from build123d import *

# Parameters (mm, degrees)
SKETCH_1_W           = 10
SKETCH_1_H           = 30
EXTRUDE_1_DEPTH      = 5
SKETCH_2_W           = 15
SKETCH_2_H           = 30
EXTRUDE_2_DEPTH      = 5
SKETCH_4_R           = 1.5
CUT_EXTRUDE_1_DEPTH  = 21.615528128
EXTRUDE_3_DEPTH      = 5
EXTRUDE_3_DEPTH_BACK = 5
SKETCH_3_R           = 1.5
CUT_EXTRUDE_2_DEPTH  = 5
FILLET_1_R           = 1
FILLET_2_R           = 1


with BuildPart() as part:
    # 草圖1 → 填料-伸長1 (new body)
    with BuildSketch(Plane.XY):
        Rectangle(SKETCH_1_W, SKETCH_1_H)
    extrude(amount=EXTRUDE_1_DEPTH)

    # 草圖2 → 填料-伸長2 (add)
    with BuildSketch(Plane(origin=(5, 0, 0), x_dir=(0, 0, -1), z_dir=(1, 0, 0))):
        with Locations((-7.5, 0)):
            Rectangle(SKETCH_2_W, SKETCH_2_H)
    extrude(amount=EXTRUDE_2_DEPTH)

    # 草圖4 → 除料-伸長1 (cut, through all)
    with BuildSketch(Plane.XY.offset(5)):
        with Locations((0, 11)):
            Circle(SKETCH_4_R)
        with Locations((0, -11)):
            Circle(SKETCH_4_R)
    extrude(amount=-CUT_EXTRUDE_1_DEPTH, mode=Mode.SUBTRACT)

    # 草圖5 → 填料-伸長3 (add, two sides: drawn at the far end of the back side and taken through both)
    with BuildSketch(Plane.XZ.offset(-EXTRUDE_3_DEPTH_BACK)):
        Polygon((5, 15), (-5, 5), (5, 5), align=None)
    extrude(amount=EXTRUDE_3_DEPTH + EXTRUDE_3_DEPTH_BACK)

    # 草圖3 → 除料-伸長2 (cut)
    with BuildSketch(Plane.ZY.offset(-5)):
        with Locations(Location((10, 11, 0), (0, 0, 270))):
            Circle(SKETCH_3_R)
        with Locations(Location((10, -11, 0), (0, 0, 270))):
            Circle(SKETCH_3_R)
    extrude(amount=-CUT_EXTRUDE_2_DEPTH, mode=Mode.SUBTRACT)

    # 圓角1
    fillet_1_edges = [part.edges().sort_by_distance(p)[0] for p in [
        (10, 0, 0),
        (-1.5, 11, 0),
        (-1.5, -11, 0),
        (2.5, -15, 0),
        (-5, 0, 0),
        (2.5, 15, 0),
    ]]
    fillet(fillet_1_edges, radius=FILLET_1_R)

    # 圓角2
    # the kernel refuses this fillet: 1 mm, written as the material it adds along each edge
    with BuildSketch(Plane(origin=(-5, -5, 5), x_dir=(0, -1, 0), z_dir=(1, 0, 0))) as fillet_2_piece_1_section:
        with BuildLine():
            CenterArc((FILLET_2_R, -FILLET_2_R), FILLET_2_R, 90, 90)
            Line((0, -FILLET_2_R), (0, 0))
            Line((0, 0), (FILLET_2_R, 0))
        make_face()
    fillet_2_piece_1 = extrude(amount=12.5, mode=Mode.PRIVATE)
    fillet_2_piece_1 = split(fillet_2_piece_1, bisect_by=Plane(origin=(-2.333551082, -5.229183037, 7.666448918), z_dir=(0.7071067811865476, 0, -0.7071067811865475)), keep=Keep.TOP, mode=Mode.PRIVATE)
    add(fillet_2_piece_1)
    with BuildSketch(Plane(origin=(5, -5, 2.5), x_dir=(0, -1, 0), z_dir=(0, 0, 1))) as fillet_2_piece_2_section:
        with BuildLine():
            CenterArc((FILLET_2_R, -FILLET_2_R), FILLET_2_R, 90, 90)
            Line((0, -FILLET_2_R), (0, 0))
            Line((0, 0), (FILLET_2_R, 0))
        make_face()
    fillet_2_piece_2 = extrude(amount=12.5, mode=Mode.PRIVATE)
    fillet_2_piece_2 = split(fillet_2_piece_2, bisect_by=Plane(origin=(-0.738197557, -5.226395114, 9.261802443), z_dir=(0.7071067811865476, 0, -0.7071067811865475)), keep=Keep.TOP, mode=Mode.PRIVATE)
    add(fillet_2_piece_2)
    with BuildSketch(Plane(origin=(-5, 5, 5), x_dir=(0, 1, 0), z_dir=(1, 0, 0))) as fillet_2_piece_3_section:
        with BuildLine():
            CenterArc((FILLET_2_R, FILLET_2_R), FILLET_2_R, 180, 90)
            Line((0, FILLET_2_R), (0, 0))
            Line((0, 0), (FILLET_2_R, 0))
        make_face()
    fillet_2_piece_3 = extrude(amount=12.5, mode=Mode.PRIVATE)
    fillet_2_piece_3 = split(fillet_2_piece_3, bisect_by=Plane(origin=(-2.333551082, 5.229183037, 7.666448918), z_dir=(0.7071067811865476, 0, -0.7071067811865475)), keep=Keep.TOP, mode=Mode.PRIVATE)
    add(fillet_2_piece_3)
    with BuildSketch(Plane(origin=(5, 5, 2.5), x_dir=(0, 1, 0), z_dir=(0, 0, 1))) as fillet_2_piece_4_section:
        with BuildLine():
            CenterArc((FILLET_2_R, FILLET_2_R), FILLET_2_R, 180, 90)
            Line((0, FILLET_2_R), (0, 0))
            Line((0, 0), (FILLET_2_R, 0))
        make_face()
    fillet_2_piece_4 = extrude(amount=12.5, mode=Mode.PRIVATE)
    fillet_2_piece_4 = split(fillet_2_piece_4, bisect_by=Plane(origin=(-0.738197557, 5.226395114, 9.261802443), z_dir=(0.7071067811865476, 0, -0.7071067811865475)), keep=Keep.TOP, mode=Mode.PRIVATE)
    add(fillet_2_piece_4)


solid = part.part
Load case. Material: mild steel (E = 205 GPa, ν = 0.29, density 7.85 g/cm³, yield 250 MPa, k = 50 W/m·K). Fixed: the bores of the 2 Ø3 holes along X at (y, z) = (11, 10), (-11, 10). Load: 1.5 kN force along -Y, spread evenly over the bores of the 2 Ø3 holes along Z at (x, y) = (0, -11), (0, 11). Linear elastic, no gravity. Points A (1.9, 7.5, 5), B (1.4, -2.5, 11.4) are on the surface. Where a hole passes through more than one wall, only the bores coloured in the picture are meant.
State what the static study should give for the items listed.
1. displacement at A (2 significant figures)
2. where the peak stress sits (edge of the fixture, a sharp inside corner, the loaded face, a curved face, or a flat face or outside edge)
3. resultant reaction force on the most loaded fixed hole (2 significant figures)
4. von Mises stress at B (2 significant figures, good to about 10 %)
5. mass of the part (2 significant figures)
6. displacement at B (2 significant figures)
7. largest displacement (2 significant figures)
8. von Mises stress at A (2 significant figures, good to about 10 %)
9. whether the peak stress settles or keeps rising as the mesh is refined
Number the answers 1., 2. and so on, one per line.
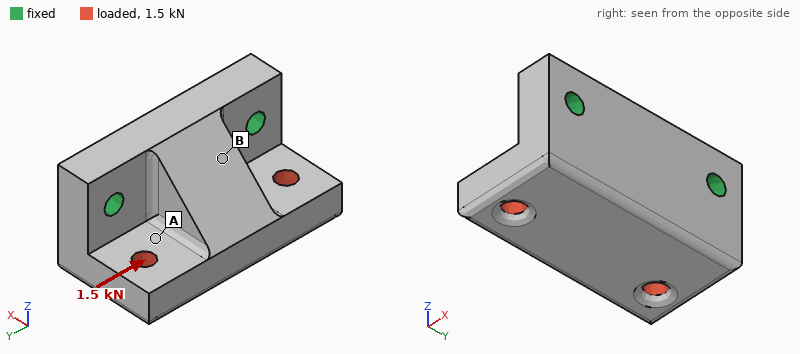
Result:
1. 2.2 µm
2. edge of the fixture
3. 1.0 kN
4. 13 MPa
5. 32 g
6. 1.1 µm
7. 4.0 µm
8. 26 MPa
9. keeps rising
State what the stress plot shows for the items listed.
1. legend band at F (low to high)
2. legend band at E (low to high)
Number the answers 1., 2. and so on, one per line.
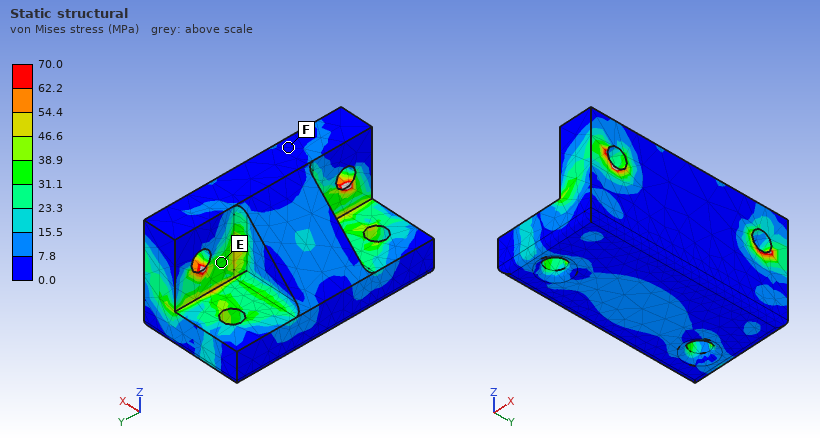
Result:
1. 0.0 to 7.8 MPa
2. 31.1 to 38.9 MPa
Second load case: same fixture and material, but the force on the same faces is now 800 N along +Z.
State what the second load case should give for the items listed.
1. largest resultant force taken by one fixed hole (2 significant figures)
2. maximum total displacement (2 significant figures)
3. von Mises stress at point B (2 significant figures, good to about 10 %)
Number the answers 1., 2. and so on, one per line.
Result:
1. 400 N
2. 10.0 µm
3. 12 MPa
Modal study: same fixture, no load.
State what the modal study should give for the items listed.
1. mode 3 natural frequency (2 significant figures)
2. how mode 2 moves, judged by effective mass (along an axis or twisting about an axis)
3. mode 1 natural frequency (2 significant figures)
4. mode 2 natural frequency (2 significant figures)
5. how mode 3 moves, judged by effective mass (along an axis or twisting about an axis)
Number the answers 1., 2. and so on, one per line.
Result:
1. 32 kHz
2. along Y
3. 13 kHz
4. 27 kHz
5. along X
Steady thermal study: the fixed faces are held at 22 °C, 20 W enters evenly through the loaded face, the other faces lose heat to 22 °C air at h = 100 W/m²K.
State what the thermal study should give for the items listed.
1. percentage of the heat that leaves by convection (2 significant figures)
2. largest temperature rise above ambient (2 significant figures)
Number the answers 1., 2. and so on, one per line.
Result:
1. 17 %
2. 42 K
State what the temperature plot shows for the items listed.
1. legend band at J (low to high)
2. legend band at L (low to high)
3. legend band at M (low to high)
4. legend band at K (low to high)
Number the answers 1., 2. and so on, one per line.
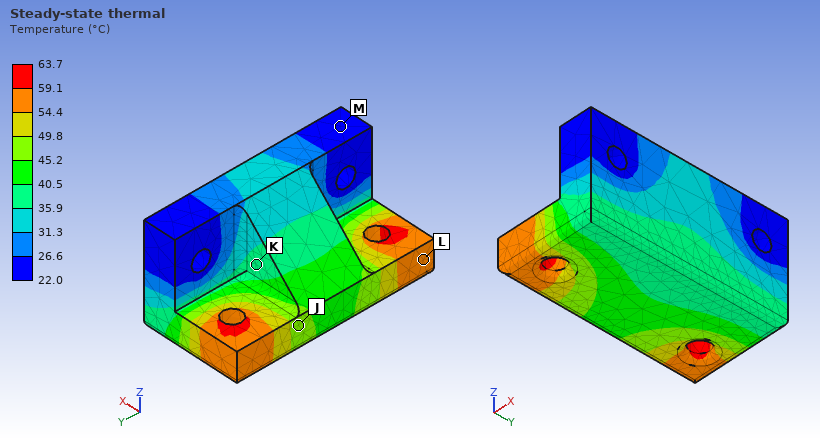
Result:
1. 45.2 to 49.8 °C
2. 54.4 to 59.1 °C
3. 22.0 to 26.6 °C
4. 35.9 to 40.5 °C
